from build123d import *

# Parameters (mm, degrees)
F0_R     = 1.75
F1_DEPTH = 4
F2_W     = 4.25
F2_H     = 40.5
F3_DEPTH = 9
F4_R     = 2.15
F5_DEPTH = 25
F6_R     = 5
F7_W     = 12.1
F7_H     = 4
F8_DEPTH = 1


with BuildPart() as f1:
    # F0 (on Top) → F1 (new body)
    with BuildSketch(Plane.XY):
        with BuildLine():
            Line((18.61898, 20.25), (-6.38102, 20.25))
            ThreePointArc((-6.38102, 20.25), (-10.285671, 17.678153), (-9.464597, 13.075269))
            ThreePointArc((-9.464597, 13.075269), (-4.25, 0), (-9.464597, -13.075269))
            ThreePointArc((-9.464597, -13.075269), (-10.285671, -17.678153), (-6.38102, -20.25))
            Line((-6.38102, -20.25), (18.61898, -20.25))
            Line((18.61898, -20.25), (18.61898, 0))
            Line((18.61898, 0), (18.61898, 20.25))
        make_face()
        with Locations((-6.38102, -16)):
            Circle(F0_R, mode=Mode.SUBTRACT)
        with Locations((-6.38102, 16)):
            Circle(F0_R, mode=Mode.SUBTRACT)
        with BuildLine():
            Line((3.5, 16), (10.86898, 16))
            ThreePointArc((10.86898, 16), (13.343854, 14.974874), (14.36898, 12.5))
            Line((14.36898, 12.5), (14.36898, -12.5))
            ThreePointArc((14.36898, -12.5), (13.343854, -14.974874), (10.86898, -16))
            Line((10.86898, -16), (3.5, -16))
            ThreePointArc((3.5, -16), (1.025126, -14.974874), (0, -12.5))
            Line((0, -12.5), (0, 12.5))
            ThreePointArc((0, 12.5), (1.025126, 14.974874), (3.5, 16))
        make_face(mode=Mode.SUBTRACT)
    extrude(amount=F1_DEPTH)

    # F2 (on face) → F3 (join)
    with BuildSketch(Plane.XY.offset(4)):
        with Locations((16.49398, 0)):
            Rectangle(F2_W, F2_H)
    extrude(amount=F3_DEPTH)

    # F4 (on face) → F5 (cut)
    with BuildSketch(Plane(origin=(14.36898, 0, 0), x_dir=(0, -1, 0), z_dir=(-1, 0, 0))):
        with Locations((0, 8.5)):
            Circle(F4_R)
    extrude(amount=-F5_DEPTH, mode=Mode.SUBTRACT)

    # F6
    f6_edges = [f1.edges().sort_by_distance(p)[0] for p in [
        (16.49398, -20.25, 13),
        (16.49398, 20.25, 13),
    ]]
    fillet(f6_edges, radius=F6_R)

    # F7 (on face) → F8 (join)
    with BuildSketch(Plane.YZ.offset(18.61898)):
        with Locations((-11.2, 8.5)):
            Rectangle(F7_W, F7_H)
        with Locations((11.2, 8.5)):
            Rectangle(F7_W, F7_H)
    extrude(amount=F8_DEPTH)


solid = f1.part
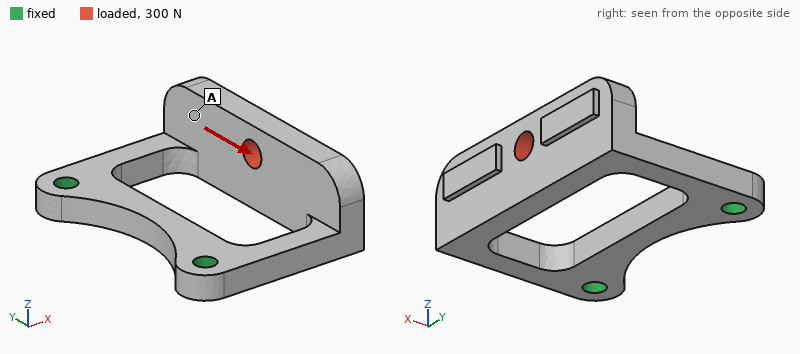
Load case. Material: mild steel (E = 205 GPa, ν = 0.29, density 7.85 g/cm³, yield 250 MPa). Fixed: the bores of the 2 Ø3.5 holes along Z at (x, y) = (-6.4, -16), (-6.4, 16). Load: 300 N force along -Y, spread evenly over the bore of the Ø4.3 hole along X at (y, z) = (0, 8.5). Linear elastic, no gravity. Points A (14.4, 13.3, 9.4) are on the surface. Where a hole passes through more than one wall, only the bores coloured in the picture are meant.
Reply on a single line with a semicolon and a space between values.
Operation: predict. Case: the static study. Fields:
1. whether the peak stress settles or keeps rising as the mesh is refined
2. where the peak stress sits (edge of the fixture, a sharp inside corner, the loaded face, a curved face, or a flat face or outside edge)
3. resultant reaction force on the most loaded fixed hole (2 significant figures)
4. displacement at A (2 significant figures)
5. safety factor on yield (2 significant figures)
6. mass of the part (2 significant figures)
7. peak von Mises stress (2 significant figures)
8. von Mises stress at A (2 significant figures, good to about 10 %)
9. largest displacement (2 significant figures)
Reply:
settles; a curved face; 200 N; 21 µm; 2.2; 30 g; 120 MPa; 18 MPa; 24 µm
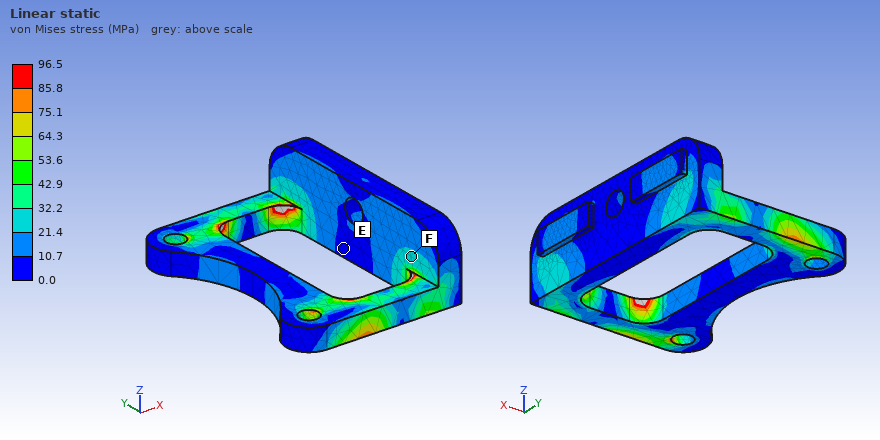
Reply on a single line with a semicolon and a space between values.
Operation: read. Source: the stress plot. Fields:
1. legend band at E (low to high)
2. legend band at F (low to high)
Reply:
0.0 to 10.7 MPa; 21.4 to 32.2 MPa
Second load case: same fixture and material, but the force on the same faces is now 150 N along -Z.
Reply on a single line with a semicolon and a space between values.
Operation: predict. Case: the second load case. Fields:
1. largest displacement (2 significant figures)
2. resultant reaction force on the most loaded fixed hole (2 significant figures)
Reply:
62 µm; 75 N
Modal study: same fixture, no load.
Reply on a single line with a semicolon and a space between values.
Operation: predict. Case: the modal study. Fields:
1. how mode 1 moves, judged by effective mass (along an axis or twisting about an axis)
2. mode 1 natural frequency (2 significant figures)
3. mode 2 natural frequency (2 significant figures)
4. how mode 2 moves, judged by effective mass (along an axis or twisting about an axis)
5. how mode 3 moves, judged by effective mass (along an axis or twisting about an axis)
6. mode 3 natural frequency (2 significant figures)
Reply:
along Z; 2000 Hz; 4400 Hz; along Y; along Y; 5800 Hz
